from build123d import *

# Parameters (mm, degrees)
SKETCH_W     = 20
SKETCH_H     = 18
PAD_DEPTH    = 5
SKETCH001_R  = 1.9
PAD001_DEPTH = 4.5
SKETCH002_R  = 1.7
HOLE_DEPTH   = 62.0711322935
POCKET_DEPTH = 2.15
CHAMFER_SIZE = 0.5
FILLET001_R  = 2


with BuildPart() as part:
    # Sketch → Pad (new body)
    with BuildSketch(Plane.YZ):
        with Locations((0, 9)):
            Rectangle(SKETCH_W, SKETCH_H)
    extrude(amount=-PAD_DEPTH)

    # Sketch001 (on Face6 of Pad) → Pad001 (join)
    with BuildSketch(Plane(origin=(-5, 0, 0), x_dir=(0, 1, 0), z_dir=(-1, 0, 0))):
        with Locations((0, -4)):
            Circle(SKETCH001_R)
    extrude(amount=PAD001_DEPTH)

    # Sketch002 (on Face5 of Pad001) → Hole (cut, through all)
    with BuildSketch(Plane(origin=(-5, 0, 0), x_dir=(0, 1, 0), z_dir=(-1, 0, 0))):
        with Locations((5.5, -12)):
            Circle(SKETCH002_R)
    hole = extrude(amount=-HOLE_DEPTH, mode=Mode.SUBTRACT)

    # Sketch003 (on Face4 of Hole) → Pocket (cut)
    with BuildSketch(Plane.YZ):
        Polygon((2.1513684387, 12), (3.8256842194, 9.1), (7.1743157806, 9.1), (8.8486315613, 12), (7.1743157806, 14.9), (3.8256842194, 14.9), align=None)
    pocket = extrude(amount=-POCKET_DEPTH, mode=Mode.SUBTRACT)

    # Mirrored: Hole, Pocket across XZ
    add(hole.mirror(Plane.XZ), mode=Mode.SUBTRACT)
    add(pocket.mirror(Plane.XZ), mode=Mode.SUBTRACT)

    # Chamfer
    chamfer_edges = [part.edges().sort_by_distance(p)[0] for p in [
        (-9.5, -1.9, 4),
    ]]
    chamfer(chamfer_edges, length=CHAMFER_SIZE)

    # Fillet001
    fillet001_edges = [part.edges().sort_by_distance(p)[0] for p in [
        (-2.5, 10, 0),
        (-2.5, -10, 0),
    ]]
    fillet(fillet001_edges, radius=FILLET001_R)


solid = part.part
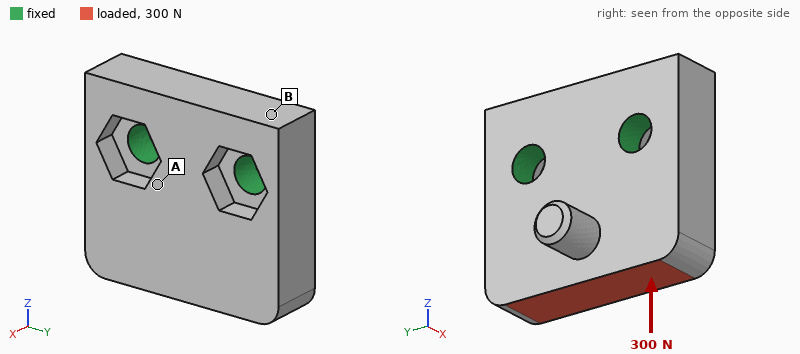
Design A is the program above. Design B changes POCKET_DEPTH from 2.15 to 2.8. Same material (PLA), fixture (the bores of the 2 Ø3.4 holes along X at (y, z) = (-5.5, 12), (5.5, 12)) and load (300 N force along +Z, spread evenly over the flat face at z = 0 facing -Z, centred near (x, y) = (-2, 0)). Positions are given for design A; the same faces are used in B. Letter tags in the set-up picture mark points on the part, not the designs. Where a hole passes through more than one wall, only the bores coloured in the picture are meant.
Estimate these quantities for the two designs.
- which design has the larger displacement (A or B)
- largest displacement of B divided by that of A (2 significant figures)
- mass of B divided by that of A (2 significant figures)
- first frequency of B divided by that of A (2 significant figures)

B
1.7
0.98
0.84
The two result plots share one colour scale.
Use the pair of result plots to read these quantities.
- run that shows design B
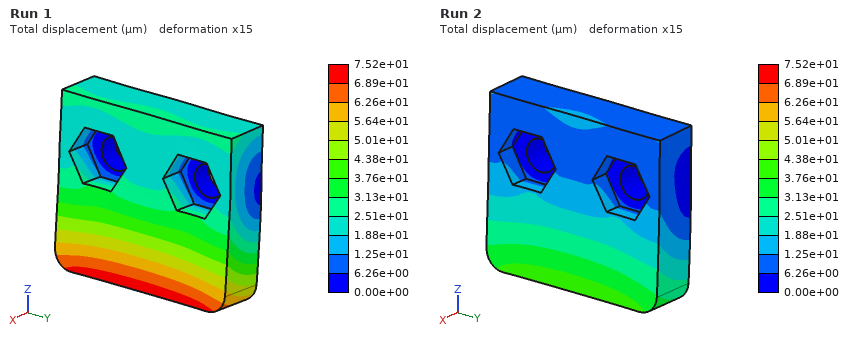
Run 1
